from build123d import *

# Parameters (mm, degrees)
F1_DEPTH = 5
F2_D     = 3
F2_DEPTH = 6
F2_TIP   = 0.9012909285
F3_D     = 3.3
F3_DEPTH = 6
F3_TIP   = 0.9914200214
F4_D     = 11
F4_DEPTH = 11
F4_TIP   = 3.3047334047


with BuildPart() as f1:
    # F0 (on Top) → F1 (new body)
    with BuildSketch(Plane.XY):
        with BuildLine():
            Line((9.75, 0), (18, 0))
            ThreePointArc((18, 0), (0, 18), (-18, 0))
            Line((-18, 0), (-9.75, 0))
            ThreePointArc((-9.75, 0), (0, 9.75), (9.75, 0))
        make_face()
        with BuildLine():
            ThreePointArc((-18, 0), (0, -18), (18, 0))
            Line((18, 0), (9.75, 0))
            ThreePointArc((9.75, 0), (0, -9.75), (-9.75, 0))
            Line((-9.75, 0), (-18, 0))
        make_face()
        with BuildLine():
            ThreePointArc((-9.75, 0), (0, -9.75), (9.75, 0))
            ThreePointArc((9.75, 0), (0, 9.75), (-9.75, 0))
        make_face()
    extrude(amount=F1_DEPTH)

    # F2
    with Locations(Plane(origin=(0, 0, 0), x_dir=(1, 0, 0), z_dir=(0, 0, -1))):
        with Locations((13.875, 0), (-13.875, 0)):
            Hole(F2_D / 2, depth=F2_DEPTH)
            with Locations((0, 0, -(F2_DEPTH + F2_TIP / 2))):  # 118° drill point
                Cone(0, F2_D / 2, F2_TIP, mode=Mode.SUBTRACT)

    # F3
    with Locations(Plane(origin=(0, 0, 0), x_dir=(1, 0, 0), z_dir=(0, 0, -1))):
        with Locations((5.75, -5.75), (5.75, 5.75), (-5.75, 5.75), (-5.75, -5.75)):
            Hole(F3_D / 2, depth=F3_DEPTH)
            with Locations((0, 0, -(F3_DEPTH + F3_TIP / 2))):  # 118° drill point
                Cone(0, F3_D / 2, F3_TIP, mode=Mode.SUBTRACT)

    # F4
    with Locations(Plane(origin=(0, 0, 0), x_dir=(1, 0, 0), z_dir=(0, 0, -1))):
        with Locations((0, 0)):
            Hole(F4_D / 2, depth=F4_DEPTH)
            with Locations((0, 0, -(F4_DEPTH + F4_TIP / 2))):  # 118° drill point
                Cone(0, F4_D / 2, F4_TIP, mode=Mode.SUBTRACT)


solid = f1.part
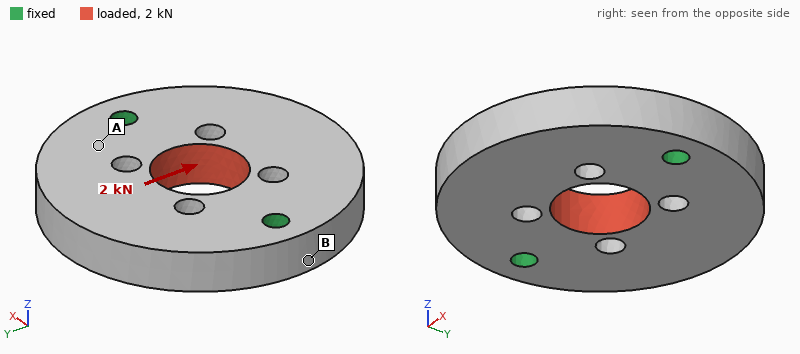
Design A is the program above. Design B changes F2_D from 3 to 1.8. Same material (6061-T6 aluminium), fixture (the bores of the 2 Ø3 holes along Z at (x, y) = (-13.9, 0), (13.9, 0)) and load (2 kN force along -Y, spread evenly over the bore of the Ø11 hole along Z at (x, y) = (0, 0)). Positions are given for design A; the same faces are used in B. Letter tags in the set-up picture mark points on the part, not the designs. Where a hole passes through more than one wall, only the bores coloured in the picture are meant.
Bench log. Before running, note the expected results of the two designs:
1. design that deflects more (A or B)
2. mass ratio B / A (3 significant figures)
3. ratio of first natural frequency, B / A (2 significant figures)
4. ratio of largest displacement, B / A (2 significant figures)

B
1.01
0.86
1.1
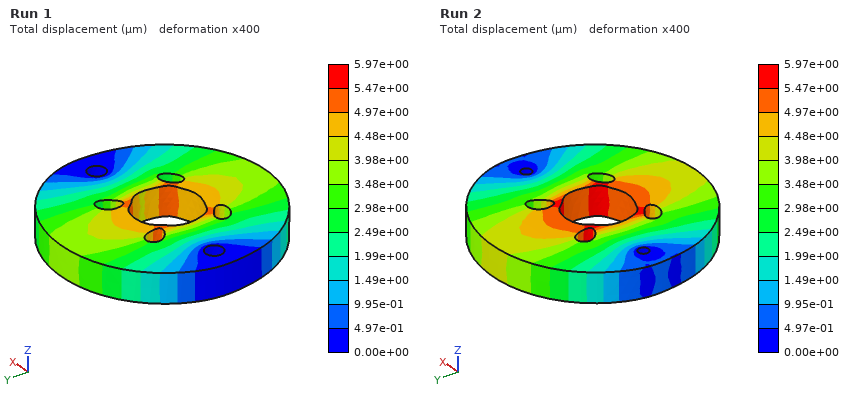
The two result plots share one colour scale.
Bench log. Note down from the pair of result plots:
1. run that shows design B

Run 2
